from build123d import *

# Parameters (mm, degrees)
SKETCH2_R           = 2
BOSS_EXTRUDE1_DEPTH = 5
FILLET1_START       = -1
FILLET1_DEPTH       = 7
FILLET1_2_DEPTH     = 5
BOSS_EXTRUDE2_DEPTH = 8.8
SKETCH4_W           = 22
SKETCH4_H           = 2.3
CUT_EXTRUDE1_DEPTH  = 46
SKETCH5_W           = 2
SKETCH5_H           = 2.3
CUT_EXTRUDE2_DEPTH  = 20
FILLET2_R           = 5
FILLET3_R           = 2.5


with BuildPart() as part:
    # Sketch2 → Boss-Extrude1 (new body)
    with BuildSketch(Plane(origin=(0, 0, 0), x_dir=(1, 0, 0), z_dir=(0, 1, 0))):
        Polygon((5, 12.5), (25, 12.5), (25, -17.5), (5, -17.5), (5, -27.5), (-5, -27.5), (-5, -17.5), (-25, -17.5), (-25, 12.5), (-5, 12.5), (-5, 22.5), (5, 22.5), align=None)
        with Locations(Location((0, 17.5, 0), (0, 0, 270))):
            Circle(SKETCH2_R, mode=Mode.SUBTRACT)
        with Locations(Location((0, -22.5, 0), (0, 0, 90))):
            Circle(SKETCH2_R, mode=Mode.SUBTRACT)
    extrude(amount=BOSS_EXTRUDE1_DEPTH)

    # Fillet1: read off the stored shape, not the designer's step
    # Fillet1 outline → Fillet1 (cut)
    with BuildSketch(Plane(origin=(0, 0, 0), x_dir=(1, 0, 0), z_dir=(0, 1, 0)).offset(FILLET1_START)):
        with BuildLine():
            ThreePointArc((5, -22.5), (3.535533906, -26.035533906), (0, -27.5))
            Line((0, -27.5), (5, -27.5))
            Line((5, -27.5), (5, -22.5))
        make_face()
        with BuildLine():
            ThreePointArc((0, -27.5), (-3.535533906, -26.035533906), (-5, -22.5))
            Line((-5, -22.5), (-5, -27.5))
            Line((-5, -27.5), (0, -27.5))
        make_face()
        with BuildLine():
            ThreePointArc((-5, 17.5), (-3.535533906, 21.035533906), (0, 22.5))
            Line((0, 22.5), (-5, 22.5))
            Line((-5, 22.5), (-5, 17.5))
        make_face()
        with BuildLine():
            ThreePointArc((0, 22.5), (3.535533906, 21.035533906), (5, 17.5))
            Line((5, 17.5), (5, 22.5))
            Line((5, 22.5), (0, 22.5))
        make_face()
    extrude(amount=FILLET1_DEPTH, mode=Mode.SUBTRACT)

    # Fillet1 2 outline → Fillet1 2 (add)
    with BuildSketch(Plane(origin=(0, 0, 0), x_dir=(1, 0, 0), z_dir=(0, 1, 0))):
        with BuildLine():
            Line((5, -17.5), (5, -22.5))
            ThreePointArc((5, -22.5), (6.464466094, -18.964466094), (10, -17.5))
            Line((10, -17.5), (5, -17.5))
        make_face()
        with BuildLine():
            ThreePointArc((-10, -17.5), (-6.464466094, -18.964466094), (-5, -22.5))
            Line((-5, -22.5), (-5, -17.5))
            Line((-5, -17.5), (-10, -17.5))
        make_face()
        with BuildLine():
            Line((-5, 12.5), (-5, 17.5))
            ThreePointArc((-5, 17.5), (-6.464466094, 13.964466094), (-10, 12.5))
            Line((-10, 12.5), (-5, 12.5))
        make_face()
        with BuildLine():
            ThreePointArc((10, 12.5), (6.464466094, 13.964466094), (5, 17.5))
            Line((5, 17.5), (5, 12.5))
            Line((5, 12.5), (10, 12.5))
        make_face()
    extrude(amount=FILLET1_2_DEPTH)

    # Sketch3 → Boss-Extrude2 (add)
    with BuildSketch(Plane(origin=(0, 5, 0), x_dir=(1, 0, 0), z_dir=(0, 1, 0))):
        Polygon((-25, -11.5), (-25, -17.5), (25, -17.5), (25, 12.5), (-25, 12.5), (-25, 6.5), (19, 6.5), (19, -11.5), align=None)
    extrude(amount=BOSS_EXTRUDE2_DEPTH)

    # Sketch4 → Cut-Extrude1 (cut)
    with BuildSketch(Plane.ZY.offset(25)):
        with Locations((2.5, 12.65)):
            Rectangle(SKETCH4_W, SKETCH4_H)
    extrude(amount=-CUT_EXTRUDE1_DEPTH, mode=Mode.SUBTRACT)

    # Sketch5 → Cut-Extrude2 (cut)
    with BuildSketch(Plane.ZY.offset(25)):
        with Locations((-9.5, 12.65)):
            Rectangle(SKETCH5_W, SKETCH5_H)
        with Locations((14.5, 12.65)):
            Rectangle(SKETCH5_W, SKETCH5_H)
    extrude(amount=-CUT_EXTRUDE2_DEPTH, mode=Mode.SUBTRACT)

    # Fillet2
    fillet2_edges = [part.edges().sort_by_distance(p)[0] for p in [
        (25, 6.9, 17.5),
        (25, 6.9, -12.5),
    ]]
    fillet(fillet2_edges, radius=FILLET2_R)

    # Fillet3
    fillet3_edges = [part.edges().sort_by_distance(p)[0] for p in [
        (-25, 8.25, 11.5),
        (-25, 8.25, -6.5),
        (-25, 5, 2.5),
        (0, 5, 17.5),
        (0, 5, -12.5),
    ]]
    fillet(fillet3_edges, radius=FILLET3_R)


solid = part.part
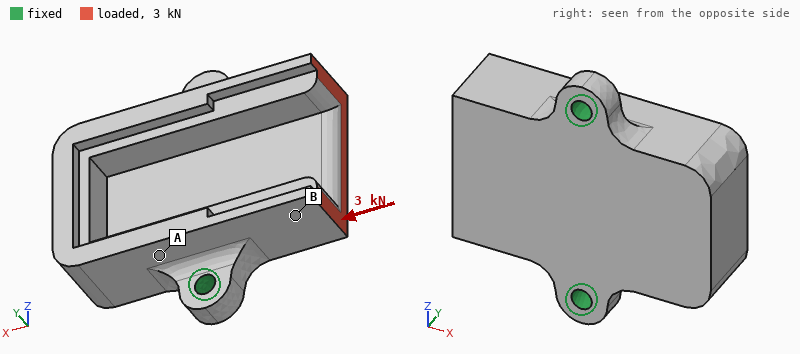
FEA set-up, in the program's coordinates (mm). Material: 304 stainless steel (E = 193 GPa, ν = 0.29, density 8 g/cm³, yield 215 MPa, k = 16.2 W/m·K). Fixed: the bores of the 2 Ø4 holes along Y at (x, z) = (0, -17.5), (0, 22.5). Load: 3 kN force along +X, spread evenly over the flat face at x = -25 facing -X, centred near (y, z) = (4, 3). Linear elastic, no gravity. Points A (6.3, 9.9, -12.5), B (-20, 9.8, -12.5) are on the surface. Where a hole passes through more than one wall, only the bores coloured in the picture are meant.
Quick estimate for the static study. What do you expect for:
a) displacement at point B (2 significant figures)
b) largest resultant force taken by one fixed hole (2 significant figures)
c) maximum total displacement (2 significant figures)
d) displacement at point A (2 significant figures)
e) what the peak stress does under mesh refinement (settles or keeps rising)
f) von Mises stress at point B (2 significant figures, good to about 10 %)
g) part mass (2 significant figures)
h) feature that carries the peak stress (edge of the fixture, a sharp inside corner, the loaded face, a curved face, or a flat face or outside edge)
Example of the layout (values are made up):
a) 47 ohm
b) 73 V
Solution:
a) 11 µm
b) 1.5 kN
c) 14 µm
d) 6.0 µm
e) keeps rising
f) 21 MPa
g) 110 g
h) edge of the fixture
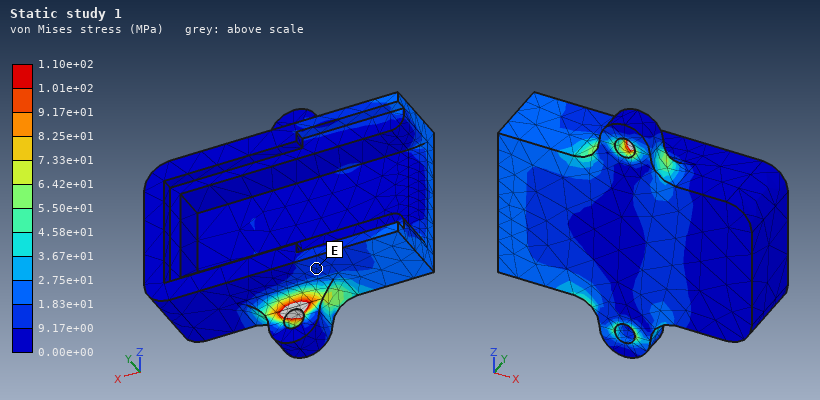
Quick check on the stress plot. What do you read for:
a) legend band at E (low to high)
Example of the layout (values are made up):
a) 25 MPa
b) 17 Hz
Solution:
a) 9.17e+00 to 1.83e+01 MPa
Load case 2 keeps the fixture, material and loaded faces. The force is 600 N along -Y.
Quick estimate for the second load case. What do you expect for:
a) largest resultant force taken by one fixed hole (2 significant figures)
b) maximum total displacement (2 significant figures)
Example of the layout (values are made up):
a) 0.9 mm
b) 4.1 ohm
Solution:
a) 310 N
b) 40 µm
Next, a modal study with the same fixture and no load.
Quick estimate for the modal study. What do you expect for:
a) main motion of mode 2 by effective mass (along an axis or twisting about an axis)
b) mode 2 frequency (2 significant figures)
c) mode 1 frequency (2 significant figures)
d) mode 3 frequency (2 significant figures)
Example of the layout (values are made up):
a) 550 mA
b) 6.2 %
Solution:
a) along Y
b) 8100 Hz
c) 3500 Hz
d) 11 kHz
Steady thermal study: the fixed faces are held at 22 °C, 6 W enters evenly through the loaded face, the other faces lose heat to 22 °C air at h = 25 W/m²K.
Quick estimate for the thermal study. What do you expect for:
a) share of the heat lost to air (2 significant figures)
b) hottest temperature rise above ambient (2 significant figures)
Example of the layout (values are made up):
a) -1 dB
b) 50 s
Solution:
a) 39 %
b) 45 K
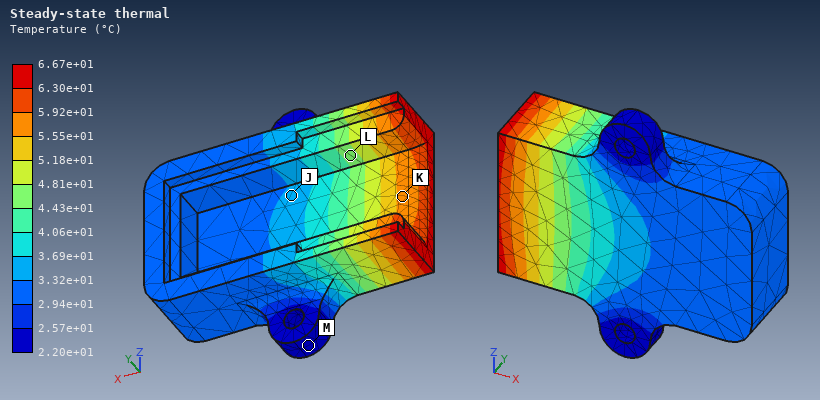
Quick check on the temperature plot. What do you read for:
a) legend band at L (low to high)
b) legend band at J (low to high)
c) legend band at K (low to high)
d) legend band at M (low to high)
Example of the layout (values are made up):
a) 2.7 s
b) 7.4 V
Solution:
a) 4.43e+01 to 4.81e+01 °C
b) 3.32e+01 to 3.69e+01 °C
c) 5.55e+01 to 5.92e+01 °C
d) 2.20e+01 to 2.57e+01 °C
